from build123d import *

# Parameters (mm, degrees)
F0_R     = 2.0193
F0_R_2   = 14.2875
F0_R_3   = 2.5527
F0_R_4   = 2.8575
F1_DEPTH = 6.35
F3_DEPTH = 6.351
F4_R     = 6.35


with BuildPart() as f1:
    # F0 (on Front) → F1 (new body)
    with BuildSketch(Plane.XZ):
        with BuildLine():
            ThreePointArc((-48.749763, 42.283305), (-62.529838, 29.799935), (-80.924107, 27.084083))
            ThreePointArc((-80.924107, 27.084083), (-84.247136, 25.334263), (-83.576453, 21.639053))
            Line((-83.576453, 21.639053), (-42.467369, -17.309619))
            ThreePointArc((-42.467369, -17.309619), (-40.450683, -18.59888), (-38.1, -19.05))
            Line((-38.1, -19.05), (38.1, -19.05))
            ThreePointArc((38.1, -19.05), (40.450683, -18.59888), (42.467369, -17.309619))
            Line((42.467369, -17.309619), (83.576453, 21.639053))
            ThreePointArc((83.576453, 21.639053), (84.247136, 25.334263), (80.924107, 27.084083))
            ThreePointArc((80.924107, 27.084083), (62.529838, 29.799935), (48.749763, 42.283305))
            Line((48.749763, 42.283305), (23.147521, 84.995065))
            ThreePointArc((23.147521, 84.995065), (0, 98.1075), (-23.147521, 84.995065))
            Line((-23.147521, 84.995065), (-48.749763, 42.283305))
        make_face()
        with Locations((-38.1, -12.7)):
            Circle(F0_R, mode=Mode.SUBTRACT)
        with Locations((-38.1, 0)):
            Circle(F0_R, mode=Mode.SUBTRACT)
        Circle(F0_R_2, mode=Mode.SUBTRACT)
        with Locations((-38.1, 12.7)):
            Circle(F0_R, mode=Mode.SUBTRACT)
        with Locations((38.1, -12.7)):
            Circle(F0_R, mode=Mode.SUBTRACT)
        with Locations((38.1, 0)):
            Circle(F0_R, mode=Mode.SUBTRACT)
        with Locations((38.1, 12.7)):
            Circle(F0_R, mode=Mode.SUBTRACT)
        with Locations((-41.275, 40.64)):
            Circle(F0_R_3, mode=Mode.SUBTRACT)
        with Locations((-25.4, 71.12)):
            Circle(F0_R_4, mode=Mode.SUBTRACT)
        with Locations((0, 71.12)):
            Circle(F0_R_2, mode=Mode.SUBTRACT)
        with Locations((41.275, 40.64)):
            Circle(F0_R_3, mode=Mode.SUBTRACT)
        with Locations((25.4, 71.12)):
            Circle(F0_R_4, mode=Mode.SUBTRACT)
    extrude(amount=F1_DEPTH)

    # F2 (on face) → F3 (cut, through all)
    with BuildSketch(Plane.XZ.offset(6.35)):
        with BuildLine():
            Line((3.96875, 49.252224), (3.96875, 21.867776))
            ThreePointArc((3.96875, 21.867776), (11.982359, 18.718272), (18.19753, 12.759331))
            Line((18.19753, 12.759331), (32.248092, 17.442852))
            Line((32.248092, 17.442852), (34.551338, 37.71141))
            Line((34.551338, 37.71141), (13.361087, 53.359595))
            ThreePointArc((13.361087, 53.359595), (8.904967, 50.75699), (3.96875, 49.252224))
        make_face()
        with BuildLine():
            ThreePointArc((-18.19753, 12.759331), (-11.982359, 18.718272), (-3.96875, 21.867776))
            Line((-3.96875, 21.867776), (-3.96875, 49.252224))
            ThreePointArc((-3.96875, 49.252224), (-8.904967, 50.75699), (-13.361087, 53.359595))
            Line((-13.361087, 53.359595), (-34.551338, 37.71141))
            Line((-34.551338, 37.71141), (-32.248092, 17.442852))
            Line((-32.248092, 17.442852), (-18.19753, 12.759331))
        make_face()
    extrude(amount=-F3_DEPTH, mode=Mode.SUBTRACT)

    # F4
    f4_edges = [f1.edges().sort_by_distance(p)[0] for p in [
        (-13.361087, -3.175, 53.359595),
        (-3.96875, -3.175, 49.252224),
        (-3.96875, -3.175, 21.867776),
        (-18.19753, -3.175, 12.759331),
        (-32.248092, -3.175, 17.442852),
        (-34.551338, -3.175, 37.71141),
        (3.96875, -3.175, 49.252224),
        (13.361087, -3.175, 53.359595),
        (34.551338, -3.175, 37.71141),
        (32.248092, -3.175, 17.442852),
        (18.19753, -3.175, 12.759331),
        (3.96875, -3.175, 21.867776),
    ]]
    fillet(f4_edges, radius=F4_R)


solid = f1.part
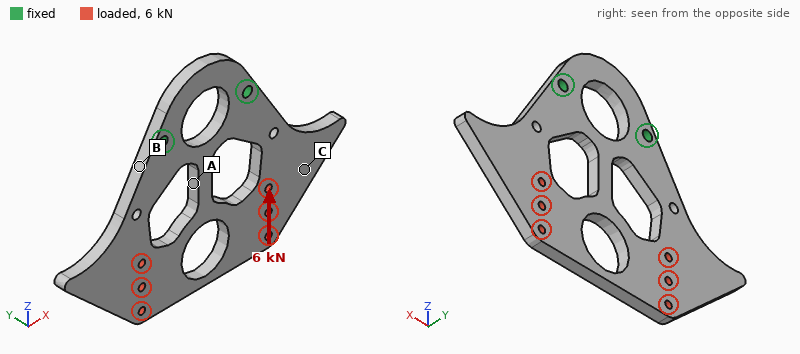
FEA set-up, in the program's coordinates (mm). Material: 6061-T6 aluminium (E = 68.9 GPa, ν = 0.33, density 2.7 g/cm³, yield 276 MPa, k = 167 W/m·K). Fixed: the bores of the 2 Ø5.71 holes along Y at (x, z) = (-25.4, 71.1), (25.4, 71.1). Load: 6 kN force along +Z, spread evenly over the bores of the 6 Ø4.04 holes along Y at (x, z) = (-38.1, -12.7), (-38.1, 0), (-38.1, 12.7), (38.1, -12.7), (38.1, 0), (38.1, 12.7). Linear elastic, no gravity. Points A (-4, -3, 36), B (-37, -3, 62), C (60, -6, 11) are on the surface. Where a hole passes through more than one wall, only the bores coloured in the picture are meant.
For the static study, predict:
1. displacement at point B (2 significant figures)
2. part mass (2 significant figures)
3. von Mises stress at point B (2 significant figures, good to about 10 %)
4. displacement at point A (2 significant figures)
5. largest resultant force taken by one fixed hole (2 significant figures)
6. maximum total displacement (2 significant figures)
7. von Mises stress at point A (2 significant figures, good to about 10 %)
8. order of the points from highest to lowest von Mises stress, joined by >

12 µm
140 g
40 MPa
15 µm
3.0 kN
47 µm
27 MPa
B > A > C
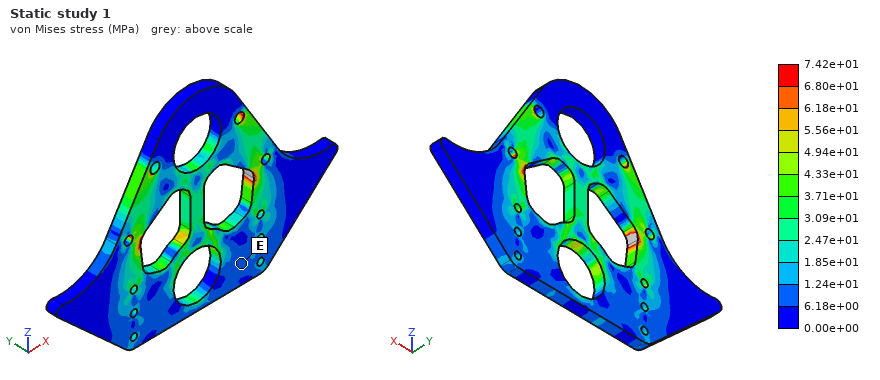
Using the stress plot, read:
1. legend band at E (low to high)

6.18e+00 to 1.24e+01 MPa
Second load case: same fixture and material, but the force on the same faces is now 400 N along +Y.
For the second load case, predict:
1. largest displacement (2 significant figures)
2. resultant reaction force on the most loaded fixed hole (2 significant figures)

1.1 mm
200 N
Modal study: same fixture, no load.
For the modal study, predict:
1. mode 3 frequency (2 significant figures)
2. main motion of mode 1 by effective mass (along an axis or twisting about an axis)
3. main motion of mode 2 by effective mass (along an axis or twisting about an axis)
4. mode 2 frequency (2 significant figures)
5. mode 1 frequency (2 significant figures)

1500 Hz
along Y
twisting about Z
700 Hz
430 Hz
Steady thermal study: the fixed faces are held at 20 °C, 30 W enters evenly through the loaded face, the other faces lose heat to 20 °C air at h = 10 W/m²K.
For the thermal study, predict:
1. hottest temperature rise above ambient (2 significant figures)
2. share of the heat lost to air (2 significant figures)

38 K
16 %
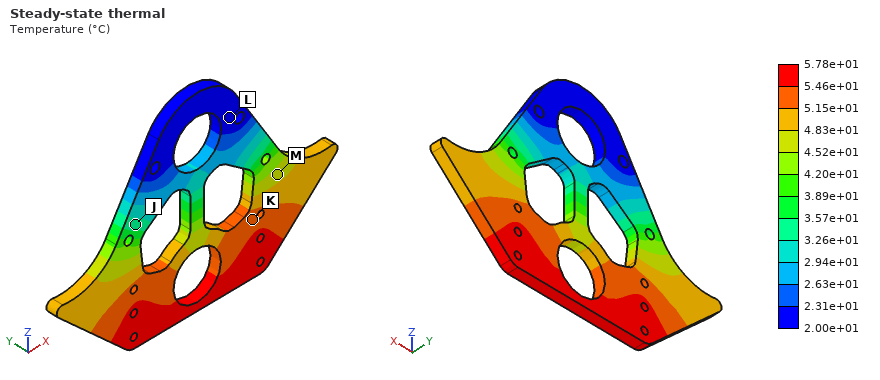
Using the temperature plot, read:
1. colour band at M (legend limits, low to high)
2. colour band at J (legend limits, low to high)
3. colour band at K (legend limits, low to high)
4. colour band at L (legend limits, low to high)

4.52e+01 to 4.83e+01 °C
3.26e+01 to 3.57e+01 °C
5.15e+01 to 5.46e+01 °C
2.00e+01 to 2.31e+01 °C
